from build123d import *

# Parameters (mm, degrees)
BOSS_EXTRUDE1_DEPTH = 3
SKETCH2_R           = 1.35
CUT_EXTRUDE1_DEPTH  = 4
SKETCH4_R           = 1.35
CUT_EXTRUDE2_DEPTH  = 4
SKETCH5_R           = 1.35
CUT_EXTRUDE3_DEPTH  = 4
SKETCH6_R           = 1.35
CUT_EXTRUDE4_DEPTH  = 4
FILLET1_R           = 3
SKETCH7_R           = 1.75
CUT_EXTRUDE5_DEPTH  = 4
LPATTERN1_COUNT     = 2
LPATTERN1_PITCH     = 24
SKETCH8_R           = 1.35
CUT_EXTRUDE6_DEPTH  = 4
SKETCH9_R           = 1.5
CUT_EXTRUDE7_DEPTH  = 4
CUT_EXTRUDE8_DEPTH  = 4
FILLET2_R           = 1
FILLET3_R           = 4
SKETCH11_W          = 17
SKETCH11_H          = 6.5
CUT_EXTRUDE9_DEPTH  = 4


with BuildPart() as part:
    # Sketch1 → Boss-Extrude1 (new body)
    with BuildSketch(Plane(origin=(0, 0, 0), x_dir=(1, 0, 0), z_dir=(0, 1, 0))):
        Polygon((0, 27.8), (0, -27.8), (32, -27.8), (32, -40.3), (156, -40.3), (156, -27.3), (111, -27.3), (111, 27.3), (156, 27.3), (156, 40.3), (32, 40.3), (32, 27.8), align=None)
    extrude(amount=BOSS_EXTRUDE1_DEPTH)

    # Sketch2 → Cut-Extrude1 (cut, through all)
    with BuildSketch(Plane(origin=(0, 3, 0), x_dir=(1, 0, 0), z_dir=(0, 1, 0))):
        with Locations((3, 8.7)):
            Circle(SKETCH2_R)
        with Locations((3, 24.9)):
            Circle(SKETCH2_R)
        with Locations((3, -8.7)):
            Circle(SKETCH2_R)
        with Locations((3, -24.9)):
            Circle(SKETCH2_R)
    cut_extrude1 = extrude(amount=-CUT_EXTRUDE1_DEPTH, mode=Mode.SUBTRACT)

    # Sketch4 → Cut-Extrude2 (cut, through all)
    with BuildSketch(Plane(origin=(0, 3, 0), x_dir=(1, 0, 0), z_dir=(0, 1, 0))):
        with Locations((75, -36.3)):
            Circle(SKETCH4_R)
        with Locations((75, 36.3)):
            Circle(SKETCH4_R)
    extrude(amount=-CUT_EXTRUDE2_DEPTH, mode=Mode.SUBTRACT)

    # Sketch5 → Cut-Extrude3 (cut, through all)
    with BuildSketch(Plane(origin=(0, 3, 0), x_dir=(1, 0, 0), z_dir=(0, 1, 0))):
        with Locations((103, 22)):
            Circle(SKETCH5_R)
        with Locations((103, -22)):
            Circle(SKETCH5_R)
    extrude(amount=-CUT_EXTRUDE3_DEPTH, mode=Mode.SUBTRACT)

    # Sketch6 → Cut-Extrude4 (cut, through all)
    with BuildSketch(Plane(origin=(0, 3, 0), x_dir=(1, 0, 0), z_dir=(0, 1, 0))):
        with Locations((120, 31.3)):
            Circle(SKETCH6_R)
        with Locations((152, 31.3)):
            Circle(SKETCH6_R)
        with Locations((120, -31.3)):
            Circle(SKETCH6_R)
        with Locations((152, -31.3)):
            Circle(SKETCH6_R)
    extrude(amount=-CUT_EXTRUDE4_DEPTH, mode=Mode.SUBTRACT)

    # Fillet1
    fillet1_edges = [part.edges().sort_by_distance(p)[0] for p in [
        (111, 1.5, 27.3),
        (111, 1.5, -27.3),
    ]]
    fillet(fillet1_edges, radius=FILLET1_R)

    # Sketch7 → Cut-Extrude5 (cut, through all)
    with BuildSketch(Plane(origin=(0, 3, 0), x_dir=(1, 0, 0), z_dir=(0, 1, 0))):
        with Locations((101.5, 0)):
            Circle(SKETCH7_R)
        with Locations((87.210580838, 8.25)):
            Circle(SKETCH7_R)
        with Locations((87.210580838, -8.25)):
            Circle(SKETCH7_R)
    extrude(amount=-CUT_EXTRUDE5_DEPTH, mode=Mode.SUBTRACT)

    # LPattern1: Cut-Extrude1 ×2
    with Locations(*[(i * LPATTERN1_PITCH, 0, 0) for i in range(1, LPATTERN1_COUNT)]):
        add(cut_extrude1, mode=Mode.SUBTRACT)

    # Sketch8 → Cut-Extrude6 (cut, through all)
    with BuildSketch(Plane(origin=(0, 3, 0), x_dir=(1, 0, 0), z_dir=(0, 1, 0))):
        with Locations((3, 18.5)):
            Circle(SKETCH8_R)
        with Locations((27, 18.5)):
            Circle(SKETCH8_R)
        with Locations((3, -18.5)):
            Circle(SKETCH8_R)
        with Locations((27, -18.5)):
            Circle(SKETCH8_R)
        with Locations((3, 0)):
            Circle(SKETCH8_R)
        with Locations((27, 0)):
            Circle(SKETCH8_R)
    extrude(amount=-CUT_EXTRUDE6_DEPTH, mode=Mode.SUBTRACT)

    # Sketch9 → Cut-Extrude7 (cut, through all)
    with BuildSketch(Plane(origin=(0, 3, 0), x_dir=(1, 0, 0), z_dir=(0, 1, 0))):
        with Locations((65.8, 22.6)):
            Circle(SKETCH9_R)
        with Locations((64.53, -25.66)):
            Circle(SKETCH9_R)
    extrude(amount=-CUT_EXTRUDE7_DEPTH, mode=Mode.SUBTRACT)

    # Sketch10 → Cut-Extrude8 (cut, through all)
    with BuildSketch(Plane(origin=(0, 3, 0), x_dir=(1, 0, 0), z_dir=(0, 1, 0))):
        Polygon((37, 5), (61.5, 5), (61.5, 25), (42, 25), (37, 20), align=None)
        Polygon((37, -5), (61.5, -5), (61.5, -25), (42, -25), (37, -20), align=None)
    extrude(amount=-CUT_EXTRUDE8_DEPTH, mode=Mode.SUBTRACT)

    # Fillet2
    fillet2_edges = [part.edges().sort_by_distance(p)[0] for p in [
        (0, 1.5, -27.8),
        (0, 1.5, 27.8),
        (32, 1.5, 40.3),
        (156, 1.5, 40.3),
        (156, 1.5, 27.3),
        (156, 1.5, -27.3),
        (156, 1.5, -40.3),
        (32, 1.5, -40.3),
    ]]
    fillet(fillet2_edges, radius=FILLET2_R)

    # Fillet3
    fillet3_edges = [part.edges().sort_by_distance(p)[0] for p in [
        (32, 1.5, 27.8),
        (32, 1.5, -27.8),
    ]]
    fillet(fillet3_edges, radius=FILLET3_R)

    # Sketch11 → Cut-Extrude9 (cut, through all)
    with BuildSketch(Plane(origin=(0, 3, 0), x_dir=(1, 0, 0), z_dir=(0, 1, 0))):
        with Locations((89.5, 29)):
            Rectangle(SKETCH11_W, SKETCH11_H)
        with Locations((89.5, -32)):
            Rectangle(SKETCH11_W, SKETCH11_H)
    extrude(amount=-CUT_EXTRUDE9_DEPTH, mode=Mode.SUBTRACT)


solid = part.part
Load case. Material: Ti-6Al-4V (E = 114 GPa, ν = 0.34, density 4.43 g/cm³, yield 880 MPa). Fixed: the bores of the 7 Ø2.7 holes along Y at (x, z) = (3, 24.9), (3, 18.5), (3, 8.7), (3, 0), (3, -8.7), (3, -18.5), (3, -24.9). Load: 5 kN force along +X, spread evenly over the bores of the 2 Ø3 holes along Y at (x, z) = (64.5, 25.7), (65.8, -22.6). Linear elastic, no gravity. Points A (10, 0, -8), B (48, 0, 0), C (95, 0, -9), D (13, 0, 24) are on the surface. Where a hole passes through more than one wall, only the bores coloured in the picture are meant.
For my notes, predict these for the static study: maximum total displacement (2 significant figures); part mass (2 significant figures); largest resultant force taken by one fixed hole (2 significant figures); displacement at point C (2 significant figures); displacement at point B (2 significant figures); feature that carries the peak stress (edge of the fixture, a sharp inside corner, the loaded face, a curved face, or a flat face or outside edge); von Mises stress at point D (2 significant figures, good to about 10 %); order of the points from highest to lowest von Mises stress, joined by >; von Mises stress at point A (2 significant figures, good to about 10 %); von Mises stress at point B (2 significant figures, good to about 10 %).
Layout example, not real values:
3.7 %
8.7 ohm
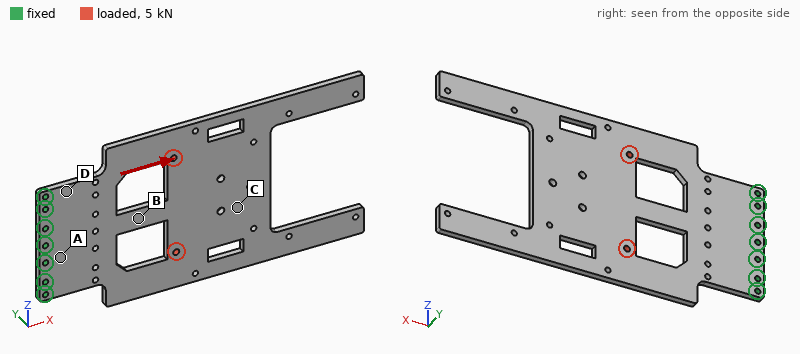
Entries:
40 µm
110 g
820 N
31 µm
16 µm
a curved face
43 MPa
B > D > A > C
23 MPa
69 MPa
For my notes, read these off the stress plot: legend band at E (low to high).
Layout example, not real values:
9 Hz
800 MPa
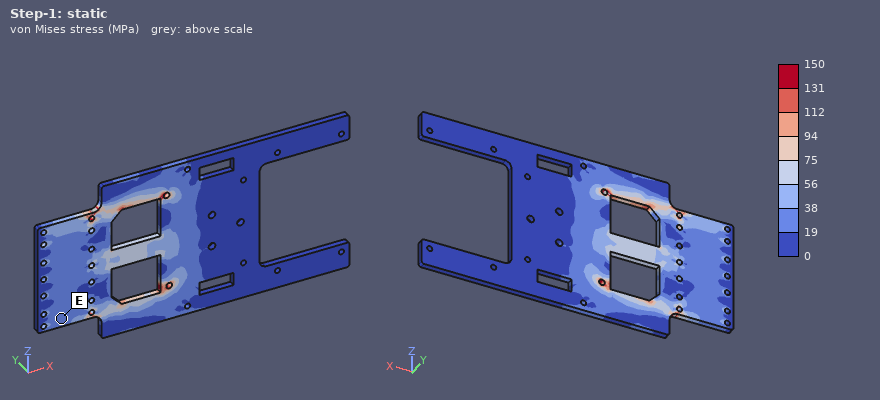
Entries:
19 to 38 MPa
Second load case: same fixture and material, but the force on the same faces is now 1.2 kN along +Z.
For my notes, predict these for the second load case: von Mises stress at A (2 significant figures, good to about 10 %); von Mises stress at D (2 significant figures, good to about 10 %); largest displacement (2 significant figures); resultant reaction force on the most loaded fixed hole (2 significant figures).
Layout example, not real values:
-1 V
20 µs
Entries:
17 MPa
39 MPa
0.18 mm
940 N
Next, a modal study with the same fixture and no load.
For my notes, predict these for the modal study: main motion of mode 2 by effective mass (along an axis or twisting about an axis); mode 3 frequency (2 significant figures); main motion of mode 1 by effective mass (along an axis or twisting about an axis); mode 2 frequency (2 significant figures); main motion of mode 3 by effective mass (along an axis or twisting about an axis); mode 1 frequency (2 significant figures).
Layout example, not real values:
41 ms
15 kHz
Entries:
twisting about X
680 Hz
along Y
340 Hz
along Y
120 Hz
